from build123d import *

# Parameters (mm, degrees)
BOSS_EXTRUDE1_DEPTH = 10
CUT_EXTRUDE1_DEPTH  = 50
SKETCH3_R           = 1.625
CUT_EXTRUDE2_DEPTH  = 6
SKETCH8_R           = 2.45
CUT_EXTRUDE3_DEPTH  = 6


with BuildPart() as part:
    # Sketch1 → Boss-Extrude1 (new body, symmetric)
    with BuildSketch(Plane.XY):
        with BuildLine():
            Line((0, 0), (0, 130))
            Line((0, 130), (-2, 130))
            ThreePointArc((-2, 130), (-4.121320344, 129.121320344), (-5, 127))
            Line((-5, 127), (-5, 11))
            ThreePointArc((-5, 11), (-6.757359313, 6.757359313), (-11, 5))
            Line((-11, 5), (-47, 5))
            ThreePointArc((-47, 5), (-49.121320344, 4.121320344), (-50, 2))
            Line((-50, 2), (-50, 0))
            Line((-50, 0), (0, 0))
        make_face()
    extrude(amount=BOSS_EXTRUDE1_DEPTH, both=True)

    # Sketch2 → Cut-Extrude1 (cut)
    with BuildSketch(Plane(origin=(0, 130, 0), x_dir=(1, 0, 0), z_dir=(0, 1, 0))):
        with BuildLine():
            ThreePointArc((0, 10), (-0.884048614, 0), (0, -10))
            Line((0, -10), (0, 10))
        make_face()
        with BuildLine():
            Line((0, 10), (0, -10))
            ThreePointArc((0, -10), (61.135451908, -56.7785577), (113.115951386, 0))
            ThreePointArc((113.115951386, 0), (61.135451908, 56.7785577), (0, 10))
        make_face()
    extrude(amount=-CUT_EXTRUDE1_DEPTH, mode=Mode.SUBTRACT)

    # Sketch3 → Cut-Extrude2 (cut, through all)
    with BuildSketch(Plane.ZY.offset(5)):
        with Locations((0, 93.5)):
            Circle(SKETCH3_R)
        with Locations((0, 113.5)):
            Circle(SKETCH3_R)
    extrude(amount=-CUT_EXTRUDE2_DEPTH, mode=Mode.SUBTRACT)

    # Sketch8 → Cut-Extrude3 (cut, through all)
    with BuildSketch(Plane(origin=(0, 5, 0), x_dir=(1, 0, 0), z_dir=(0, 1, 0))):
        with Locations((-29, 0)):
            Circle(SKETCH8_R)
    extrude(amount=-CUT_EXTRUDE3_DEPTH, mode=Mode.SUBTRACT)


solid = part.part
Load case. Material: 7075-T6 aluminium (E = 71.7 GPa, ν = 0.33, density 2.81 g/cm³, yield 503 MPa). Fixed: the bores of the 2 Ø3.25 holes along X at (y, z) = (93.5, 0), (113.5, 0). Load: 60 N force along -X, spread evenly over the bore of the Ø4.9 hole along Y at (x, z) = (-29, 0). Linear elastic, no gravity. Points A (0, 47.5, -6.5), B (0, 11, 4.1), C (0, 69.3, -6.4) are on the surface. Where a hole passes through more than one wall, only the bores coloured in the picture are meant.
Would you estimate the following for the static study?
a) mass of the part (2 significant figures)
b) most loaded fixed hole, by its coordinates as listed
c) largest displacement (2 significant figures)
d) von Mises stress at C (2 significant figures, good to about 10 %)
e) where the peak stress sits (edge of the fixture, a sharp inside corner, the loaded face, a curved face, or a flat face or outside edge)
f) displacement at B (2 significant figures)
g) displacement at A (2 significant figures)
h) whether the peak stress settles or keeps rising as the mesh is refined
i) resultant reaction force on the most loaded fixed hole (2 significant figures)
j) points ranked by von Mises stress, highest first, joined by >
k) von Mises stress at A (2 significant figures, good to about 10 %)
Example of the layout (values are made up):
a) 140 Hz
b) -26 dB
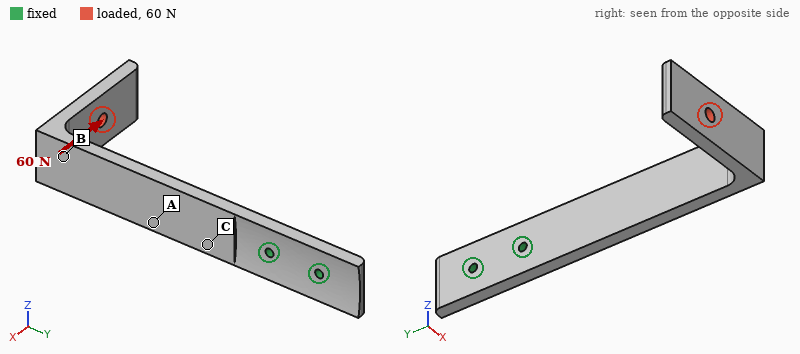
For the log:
a) 47 g
b) (93.5, 0)
c) 1.6 mm
d) 48 MPa
e) edge of the fixture
f) 1.1 mm
g) 0.42 mm
h) keeps rising
i) 170 N
j) C > A > B
k) 32 MPa
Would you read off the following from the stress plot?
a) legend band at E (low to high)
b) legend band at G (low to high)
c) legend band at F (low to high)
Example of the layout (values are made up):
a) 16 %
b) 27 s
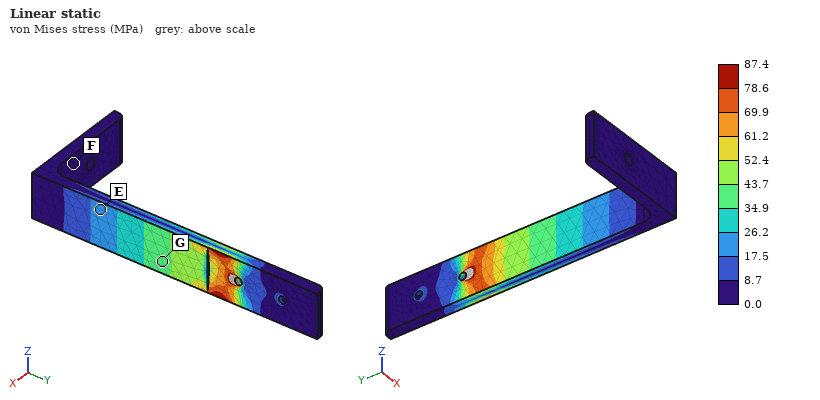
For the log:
a) 17.5 to 26.2 MPa
b) 34.9 to 43.7 MPa
c) 0.0 to 8.7 MPa
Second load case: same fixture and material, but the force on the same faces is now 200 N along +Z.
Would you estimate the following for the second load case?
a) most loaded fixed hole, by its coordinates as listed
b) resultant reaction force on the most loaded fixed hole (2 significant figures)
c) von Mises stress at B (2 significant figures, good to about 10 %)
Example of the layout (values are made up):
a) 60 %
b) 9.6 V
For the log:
a) (93.5, 0)
b) 930 N
c) 41 MPa
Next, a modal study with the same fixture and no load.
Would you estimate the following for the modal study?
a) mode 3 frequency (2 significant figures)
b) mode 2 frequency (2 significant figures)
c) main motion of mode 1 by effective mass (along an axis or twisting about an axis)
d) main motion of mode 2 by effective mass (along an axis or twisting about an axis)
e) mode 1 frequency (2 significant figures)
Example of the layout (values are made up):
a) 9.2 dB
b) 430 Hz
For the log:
a) 1100 Hz
b) 600 Hz
c) along X
d) along Z
e) 240 Hz
